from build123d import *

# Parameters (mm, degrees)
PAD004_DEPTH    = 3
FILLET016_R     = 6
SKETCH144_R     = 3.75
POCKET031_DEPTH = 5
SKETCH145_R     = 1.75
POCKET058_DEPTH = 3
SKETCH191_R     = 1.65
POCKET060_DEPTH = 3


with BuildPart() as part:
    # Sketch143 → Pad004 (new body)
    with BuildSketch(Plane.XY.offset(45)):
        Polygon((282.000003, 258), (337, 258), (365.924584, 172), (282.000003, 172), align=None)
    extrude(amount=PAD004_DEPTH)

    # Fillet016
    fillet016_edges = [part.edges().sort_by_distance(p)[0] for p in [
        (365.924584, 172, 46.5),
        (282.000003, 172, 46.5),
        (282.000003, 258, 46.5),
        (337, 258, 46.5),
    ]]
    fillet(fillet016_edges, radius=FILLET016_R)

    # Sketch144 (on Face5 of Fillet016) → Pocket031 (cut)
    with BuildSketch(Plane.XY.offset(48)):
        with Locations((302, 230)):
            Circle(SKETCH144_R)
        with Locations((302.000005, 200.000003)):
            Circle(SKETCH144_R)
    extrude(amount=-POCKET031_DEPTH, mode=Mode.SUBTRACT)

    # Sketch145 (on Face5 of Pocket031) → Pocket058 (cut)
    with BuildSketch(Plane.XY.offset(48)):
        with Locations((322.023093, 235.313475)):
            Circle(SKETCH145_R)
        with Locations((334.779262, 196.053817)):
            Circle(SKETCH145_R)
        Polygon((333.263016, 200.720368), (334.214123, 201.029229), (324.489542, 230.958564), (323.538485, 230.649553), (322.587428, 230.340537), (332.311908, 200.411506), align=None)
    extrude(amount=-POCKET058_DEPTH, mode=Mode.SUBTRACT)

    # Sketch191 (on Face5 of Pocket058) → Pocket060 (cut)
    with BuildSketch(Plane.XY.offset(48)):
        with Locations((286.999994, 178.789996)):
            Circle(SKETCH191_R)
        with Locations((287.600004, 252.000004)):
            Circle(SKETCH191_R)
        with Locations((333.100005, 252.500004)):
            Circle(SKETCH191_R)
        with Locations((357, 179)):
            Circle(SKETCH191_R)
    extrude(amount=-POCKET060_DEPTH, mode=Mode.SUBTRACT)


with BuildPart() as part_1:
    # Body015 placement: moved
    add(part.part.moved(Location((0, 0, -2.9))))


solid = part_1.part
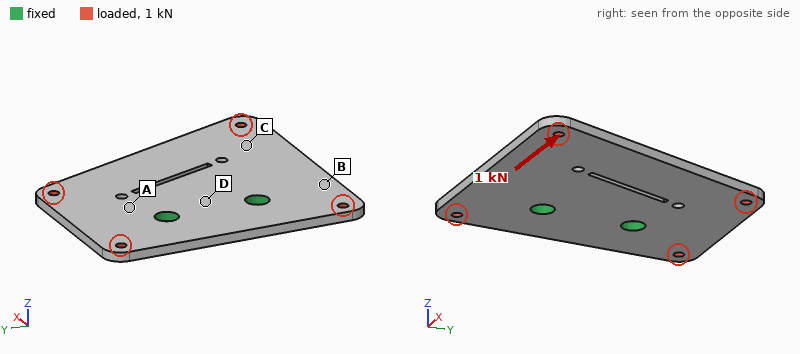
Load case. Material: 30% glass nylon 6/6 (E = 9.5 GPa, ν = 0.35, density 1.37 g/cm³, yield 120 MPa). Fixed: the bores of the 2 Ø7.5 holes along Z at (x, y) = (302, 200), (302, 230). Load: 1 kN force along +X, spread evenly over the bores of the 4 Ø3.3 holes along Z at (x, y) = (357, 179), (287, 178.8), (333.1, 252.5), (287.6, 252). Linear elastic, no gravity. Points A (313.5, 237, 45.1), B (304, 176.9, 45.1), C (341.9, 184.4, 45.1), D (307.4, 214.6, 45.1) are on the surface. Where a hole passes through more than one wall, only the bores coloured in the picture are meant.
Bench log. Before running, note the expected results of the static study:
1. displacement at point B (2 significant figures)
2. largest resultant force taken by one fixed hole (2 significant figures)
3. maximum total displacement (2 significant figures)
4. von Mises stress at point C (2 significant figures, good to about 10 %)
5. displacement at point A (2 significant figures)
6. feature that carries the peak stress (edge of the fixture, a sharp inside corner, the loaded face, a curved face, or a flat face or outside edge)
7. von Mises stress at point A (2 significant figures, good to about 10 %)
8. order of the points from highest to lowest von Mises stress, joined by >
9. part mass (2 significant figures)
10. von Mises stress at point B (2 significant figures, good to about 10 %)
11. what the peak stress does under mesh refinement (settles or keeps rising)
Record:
27 µm
510 N
49 µm
5.0 MPa
13 µm
edge of the fixture
7.8 MPa
A > C > B > D
24 g
3.2 MPa
keeps rising
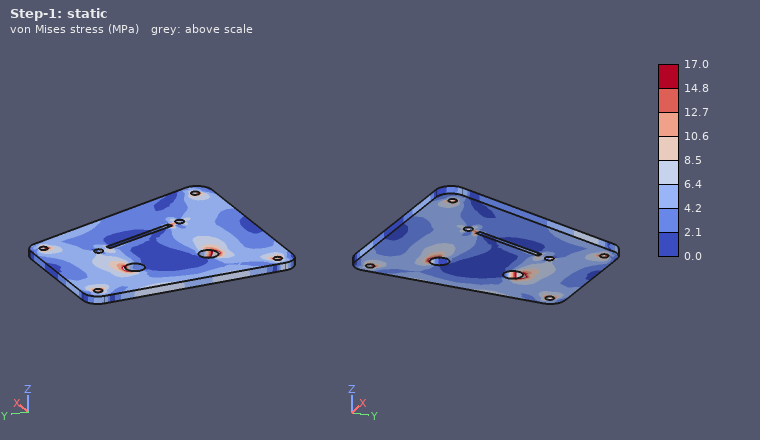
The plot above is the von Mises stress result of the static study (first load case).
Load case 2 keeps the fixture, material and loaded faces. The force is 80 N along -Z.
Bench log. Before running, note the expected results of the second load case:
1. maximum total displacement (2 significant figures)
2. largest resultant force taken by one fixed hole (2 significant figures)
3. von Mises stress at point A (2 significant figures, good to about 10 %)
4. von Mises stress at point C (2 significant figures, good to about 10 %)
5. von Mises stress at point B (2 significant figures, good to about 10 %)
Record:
1.3 mm
41 N
9.4 MPa
5.6 MPa
8.7 MPa
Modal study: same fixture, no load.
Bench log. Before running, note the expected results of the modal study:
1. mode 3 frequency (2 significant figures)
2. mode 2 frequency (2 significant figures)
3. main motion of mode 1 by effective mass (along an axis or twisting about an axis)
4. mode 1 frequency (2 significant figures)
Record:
1500 Hz
860 Hz
along Z
450 Hz
